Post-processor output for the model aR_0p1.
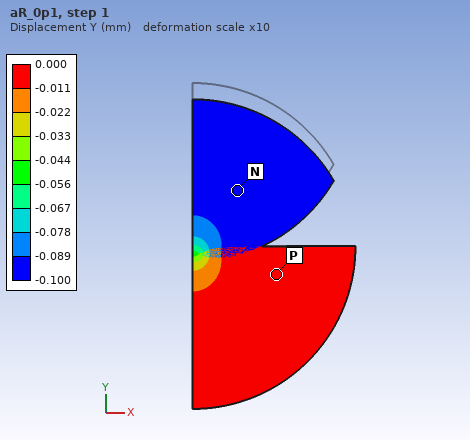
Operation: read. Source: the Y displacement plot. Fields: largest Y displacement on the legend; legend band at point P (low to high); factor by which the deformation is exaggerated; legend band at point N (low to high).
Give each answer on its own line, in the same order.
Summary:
0.000 mm
-0.011 to 0.000 mm
10
-0.100 to -0.089 mm
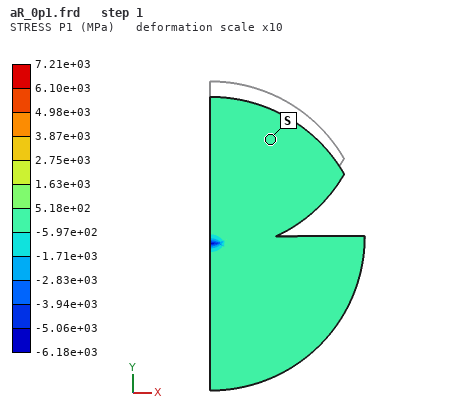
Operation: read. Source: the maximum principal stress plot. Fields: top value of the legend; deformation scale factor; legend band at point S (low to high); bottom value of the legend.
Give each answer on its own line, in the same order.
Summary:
7.21e+03 MPa
10
-5.97e+02 to 5.18e+02 MPa
-6.18e+03 MPa
